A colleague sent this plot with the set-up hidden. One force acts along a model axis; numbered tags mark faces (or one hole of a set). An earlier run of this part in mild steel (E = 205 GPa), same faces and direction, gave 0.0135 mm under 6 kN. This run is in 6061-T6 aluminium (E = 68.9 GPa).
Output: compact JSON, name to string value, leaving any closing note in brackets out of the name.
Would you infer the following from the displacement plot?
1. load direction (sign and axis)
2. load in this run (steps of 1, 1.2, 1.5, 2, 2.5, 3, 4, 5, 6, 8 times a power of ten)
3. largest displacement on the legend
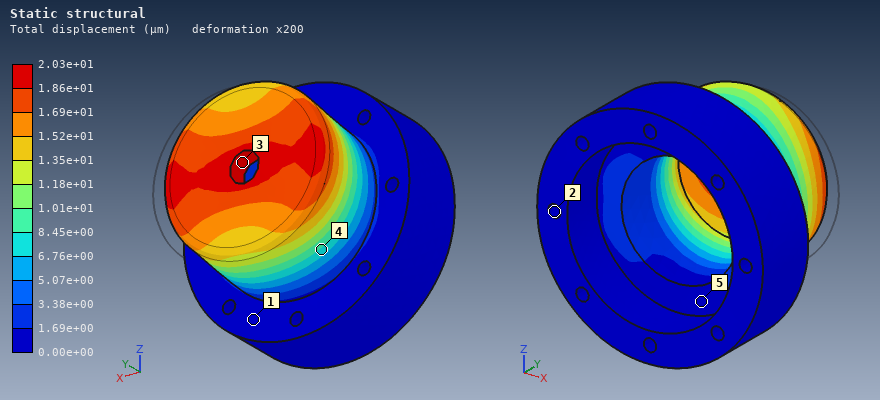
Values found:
{"load direction": "-X", "load in this run": "3 kN", "largest displacement on the legend": "2.03e+01 µm"}
